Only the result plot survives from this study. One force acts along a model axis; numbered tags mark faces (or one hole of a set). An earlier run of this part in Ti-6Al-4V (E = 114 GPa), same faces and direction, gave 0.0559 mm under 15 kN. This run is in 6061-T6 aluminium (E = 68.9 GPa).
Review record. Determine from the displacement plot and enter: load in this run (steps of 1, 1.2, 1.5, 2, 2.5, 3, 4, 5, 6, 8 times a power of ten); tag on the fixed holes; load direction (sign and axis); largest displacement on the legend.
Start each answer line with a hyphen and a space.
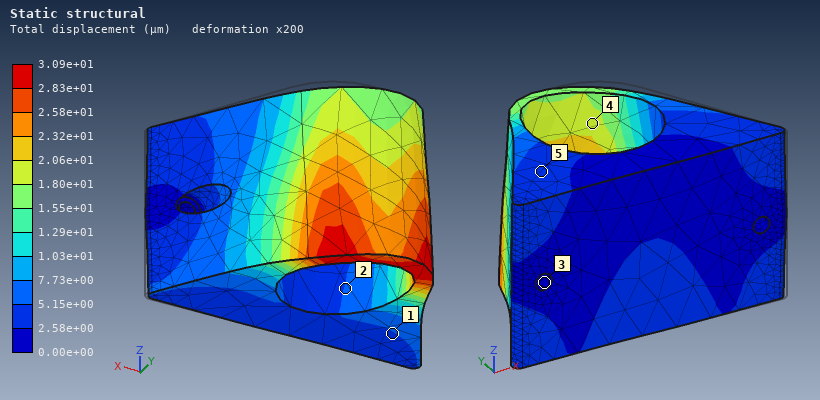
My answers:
- 5 kN
- 3
- -X
- 3.09e+01 µm
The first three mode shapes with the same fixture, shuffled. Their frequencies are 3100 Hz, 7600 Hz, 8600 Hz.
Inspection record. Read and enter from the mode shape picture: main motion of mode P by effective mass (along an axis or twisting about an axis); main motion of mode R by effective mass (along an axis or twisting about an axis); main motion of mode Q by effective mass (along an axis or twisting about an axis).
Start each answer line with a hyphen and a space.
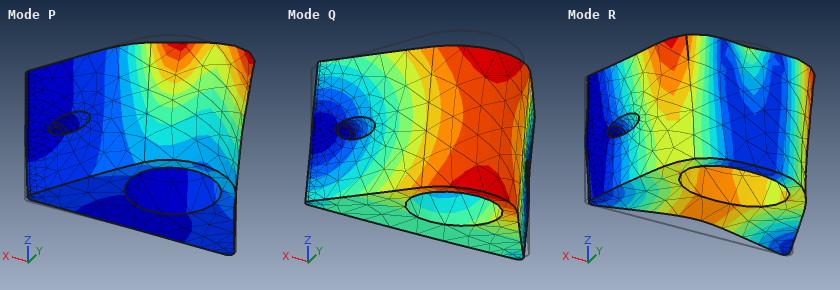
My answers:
- along X
- along Y
- along Z
